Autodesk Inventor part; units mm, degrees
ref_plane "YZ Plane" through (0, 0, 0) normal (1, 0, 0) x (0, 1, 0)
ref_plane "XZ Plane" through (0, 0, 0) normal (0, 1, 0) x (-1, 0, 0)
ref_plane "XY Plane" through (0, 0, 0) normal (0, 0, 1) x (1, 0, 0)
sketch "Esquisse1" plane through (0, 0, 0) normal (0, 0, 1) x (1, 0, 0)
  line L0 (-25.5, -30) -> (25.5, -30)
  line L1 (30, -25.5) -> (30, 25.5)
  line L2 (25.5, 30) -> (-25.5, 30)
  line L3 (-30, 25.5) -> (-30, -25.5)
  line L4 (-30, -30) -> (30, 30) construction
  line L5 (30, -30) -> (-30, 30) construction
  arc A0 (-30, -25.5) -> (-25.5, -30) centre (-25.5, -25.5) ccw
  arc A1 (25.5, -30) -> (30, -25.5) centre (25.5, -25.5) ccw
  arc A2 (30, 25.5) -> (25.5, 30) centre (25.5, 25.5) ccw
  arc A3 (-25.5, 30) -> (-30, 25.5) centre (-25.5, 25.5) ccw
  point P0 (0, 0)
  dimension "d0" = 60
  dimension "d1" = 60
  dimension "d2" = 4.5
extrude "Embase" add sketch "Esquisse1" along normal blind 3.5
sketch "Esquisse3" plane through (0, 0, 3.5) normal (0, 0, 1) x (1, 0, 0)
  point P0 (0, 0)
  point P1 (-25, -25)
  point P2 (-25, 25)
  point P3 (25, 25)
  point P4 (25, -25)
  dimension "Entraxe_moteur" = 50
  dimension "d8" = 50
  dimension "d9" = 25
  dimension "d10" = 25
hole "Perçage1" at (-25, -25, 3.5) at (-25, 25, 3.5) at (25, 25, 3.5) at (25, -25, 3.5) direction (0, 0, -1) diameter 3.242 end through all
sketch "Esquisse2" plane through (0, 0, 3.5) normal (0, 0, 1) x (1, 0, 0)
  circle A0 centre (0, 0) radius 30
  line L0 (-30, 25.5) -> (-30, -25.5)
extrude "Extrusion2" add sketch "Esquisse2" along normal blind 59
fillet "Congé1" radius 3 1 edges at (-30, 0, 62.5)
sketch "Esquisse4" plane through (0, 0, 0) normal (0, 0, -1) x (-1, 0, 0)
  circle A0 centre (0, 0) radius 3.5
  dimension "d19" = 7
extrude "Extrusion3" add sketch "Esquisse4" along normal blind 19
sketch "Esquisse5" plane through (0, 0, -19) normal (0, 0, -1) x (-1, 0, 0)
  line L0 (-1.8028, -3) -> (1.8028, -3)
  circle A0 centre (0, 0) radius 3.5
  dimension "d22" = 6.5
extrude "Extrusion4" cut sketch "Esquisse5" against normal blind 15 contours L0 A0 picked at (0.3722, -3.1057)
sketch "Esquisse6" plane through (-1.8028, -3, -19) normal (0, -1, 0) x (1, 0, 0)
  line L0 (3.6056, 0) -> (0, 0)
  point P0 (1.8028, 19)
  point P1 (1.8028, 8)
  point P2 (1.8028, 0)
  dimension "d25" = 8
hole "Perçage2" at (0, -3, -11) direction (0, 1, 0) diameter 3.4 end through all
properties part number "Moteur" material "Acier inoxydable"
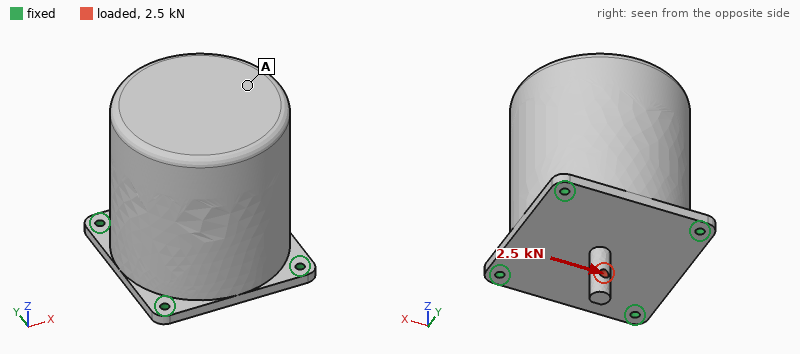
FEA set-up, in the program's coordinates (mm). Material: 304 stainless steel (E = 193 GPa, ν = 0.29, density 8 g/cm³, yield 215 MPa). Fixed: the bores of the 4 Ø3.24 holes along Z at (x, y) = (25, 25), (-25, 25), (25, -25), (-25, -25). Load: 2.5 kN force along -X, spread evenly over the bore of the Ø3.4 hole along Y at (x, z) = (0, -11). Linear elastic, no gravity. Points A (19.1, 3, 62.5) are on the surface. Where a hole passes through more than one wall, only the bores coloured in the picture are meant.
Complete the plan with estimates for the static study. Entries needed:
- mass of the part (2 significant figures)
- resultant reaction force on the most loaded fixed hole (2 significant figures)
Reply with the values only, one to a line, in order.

1.4 kg
720 N
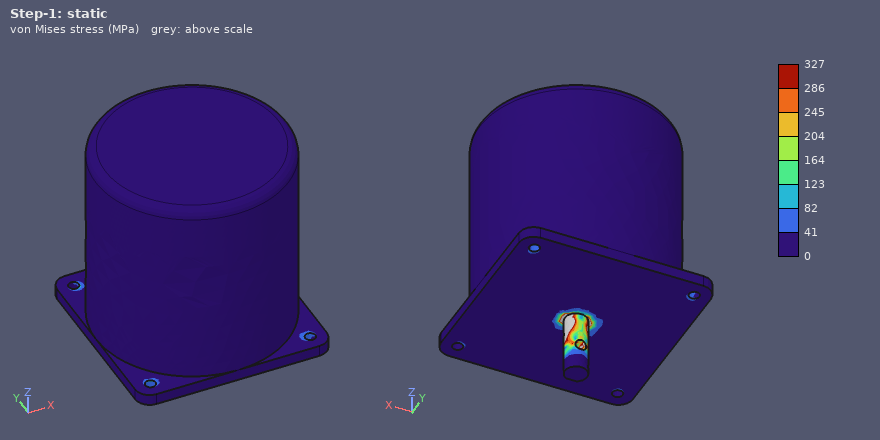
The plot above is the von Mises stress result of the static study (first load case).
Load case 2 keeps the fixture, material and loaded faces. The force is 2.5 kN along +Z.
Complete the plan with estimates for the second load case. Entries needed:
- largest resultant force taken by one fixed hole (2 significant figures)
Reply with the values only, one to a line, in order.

690 N
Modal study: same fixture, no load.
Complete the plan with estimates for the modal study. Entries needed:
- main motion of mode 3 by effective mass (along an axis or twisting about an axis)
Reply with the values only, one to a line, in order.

along Z
